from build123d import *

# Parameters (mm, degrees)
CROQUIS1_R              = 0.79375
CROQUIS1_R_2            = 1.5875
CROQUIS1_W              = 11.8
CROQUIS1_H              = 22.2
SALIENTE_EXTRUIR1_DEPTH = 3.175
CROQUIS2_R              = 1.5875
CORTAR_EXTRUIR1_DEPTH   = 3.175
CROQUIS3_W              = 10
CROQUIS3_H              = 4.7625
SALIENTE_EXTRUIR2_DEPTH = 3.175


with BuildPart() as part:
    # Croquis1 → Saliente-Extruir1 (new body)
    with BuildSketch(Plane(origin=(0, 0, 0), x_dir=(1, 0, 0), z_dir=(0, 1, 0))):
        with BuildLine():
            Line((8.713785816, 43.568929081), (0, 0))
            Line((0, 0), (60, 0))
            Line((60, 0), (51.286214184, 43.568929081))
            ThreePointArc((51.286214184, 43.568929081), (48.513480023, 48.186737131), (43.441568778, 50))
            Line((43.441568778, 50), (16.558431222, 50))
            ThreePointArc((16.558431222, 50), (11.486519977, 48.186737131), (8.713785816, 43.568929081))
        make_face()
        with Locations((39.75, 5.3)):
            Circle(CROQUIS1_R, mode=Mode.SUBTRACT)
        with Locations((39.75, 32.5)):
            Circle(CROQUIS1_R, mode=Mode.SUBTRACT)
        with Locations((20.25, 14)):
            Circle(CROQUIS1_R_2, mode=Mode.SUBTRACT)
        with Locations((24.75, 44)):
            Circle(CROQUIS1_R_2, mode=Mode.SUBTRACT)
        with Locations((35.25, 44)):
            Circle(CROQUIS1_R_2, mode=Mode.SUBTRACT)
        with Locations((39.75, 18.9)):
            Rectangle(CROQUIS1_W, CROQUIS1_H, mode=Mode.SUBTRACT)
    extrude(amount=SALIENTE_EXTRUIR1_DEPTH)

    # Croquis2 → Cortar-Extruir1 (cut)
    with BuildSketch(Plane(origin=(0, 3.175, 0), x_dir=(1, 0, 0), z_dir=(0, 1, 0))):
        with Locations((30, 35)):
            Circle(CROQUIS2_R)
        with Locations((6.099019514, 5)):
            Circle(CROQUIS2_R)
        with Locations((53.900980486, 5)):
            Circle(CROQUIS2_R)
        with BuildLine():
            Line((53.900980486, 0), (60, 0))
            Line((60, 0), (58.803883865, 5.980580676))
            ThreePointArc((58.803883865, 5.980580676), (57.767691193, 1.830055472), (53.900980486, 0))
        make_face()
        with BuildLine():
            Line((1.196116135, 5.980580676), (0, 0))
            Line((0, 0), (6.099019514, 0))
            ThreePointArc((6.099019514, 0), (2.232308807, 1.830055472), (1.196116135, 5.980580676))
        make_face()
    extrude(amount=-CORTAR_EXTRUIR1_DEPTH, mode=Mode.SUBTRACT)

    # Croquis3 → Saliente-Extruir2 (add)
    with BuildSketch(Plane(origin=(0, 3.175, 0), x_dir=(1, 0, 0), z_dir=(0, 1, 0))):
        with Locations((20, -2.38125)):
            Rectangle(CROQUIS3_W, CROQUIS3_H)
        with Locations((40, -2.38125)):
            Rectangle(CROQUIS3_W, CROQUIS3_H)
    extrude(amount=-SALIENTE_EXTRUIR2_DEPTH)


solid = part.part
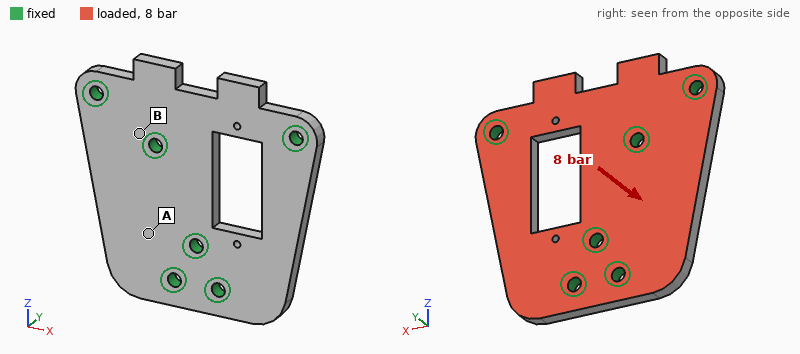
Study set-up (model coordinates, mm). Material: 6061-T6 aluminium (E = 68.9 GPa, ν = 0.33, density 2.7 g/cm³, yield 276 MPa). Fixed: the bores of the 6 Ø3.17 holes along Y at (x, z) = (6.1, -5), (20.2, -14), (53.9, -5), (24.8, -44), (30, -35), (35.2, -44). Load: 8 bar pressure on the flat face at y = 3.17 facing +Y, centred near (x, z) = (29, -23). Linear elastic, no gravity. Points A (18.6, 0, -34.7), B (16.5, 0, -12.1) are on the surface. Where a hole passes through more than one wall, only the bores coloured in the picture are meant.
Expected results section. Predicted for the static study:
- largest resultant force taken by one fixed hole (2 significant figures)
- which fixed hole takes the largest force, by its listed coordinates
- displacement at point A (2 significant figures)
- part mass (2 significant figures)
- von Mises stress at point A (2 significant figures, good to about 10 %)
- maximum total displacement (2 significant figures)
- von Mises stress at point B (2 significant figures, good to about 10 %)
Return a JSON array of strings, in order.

["510 N", "(20.2, -14)", "14 µm", "19 g", "17 MPa", "54 µm", "35 MPa"]
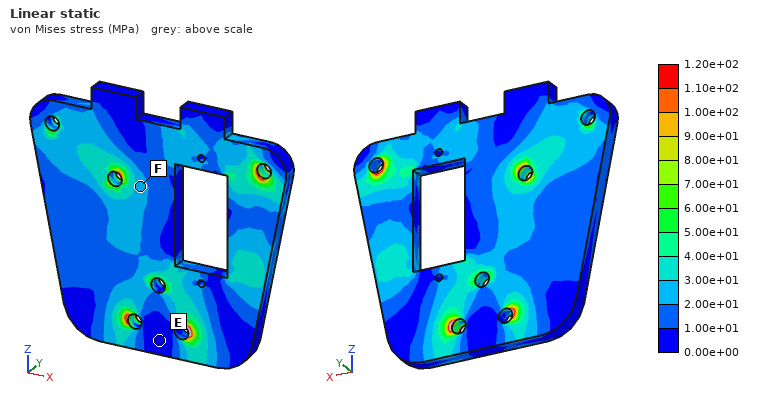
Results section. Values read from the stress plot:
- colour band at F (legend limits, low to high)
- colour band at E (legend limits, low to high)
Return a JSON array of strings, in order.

["2.00e+01 to 3.00e+01 MPa", "0.00e+00 to 1.00e+01 MPa"]
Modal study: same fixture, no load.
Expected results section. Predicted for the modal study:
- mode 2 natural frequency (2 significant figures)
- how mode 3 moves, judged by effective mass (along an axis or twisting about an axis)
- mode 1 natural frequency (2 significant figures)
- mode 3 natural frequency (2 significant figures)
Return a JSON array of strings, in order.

["9300 Hz", "along Y", "8200 Hz", "10 kHz"]
